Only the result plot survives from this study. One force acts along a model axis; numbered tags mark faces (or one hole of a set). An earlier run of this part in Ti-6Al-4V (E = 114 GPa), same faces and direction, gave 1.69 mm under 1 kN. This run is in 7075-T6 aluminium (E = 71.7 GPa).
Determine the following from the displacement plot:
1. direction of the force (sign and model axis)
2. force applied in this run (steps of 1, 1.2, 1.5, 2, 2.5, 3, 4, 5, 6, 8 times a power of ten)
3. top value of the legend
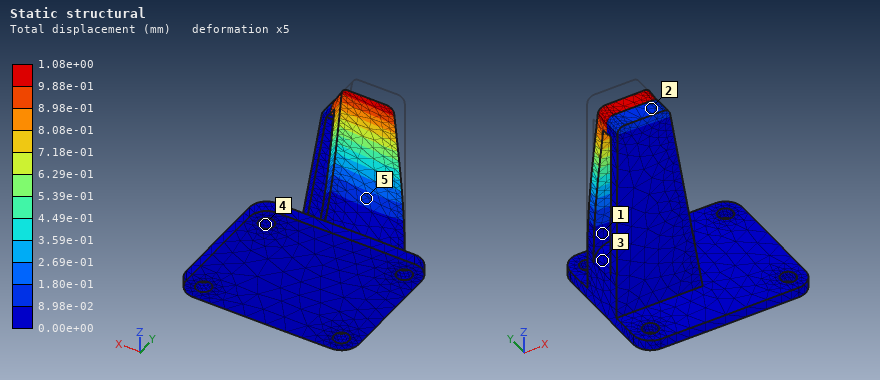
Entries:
-Y
400 N
1.08e+00 mm
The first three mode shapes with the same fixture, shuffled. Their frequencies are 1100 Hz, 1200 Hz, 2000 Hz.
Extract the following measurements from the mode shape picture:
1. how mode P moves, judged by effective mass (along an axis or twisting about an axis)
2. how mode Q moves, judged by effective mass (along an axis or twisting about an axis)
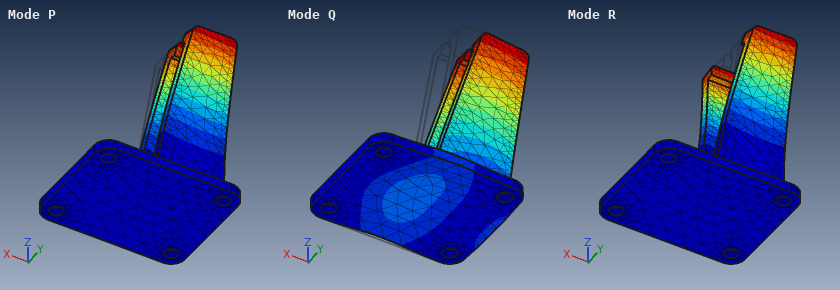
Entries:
along Y
along X
